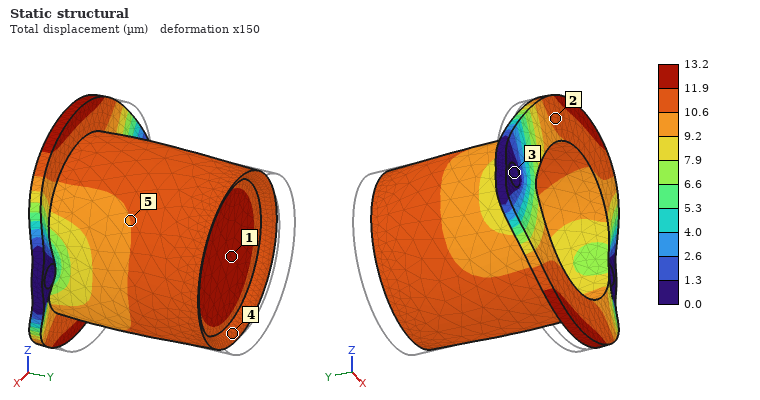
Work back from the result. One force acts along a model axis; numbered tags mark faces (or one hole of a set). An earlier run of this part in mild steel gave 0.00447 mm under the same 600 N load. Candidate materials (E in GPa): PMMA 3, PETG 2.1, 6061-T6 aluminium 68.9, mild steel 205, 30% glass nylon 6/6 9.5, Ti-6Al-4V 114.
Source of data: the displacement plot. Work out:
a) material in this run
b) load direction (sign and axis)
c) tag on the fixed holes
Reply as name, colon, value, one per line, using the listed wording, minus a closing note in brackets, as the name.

material in this run: 6061-T6 aluminium
load direction: -Y
tag on the fixed holes: 3
